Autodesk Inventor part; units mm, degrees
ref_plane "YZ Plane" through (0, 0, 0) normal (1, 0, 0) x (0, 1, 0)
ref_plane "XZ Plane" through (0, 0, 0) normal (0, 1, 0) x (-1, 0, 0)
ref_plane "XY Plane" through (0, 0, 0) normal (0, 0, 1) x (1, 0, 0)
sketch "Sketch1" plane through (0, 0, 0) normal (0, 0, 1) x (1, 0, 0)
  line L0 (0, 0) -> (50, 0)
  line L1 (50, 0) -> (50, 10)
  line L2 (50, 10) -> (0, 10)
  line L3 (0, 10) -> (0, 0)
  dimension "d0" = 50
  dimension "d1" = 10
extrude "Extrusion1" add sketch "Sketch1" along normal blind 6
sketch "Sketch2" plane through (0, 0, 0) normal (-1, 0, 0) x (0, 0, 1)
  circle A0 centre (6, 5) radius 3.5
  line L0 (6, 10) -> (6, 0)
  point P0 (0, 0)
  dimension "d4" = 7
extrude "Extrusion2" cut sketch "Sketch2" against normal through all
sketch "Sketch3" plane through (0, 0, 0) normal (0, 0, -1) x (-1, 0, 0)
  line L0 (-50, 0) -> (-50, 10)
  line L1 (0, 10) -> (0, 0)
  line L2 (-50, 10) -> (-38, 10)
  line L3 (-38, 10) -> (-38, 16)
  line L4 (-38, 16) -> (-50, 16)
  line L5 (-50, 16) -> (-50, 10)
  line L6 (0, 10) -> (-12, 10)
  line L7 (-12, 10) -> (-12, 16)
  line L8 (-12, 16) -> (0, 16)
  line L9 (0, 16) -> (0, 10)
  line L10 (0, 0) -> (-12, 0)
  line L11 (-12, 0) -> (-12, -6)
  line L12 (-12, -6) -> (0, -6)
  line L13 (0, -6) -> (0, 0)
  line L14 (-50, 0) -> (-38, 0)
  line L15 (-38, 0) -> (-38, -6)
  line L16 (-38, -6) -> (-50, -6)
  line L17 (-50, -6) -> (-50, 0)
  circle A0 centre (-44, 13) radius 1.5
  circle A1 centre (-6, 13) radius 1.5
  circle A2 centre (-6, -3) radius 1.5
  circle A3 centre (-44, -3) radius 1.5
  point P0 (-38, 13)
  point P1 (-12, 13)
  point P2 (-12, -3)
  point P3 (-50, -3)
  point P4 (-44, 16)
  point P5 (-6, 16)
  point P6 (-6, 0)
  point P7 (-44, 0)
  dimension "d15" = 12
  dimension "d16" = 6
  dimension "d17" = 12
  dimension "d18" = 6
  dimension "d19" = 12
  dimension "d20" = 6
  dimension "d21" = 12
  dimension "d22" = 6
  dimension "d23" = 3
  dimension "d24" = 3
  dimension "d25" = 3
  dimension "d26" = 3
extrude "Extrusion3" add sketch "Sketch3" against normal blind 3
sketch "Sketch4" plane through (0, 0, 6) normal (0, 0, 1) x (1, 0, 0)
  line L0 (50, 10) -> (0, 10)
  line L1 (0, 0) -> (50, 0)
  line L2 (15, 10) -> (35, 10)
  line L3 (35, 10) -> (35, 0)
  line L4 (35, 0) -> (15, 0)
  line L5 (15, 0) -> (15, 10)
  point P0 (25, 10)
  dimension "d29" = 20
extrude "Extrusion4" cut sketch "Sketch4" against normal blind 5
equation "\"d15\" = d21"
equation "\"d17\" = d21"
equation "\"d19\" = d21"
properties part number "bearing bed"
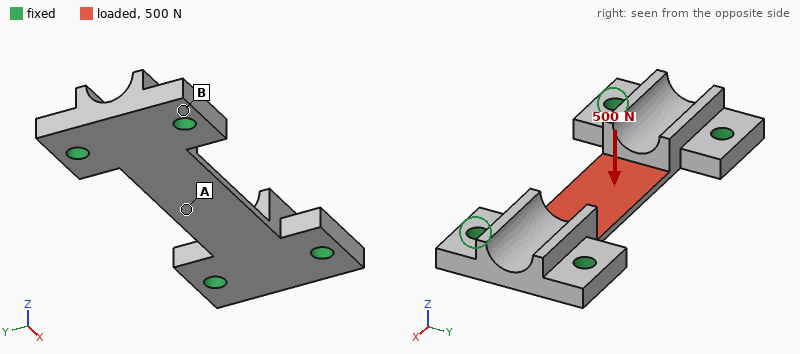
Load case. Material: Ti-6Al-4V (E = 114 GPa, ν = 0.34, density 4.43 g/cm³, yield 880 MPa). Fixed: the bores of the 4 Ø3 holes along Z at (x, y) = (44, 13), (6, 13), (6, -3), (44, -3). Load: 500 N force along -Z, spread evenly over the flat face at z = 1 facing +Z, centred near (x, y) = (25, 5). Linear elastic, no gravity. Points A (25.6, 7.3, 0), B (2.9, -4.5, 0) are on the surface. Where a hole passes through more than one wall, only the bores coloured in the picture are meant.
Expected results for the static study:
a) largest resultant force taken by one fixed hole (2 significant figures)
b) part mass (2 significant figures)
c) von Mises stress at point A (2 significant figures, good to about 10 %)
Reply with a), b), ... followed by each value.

a) 190 N
b) 9.8 g
c) 290 MPa
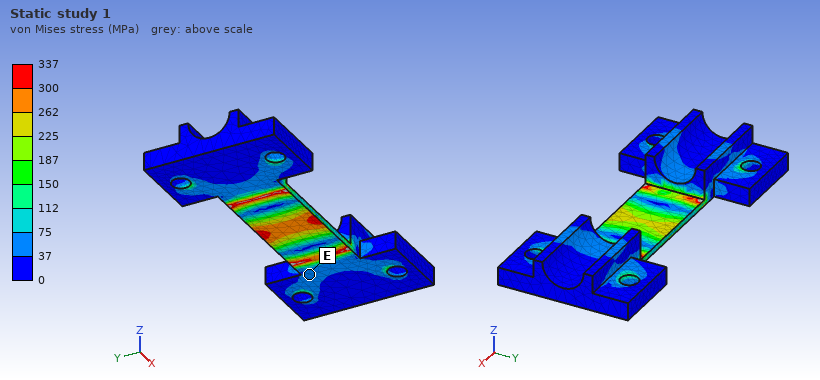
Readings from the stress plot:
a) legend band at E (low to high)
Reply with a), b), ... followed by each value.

a) 37 to 75 MPa
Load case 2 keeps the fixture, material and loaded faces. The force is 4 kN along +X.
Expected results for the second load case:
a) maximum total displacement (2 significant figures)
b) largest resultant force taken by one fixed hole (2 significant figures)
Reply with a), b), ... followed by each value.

a) 31 µm
b) 1.1 kN
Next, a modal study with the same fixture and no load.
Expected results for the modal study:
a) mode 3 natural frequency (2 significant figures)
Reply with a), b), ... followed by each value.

a) 22 kHz
